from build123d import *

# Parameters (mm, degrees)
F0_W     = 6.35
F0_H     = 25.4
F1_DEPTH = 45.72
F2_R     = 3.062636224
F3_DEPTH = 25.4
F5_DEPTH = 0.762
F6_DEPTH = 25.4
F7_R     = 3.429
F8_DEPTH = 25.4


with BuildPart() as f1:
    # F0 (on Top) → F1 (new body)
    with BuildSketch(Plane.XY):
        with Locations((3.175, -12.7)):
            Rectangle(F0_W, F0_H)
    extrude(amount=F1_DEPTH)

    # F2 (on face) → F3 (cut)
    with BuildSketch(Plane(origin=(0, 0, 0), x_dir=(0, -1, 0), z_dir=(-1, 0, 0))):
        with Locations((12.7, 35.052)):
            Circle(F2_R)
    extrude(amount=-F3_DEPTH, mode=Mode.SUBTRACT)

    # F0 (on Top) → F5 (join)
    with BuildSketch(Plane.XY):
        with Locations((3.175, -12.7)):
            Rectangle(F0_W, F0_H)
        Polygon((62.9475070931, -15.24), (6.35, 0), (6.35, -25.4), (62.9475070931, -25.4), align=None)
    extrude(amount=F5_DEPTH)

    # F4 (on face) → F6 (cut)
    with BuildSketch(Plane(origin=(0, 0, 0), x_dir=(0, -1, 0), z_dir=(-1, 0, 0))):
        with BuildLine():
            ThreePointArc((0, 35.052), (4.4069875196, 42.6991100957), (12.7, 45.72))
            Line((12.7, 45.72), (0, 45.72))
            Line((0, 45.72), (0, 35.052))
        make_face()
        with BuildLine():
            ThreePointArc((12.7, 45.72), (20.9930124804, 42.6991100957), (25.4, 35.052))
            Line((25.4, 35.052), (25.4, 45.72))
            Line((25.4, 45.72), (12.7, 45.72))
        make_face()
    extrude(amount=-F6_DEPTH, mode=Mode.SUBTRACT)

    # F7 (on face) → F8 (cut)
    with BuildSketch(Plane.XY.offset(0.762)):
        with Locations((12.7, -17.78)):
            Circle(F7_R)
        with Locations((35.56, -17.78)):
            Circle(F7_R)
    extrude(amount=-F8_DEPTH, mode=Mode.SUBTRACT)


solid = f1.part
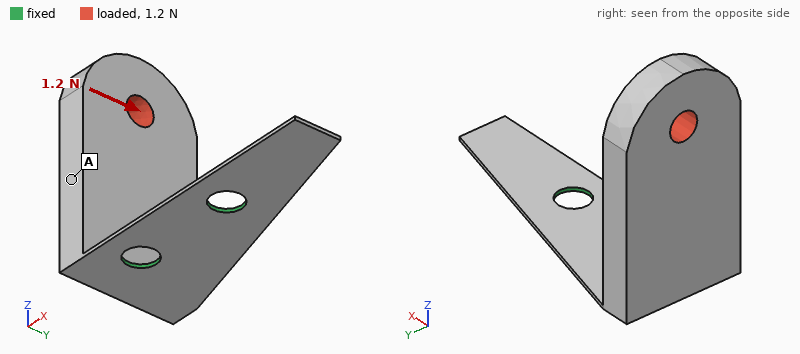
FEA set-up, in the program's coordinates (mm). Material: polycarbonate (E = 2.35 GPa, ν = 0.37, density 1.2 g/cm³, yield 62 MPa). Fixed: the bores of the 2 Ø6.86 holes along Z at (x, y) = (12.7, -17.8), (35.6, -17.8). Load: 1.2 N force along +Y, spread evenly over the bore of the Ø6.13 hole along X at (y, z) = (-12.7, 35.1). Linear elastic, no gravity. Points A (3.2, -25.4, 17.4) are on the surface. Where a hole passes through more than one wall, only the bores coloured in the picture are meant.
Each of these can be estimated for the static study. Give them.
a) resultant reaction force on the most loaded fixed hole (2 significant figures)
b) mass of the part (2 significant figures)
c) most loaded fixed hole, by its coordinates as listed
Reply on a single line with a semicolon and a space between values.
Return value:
1.3 N; 9.0 g; (12.7, -17.8)
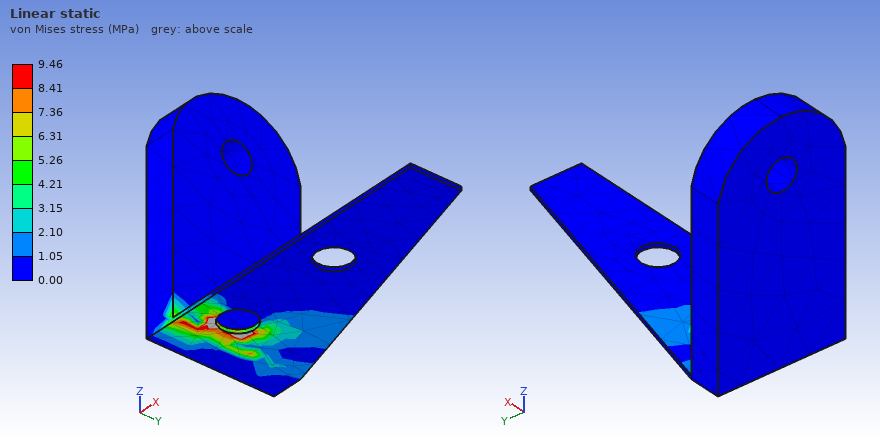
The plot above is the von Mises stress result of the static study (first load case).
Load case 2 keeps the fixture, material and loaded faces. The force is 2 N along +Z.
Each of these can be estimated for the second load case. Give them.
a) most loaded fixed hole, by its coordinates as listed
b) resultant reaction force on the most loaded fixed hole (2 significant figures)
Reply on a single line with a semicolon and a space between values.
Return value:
(12.7, -17.8); 2.0 N
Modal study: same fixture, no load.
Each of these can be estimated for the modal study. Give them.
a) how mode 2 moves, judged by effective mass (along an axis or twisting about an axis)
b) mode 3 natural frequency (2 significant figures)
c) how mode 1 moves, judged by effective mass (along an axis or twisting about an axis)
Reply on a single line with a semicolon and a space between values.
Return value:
along Y; 330 Hz; along X
